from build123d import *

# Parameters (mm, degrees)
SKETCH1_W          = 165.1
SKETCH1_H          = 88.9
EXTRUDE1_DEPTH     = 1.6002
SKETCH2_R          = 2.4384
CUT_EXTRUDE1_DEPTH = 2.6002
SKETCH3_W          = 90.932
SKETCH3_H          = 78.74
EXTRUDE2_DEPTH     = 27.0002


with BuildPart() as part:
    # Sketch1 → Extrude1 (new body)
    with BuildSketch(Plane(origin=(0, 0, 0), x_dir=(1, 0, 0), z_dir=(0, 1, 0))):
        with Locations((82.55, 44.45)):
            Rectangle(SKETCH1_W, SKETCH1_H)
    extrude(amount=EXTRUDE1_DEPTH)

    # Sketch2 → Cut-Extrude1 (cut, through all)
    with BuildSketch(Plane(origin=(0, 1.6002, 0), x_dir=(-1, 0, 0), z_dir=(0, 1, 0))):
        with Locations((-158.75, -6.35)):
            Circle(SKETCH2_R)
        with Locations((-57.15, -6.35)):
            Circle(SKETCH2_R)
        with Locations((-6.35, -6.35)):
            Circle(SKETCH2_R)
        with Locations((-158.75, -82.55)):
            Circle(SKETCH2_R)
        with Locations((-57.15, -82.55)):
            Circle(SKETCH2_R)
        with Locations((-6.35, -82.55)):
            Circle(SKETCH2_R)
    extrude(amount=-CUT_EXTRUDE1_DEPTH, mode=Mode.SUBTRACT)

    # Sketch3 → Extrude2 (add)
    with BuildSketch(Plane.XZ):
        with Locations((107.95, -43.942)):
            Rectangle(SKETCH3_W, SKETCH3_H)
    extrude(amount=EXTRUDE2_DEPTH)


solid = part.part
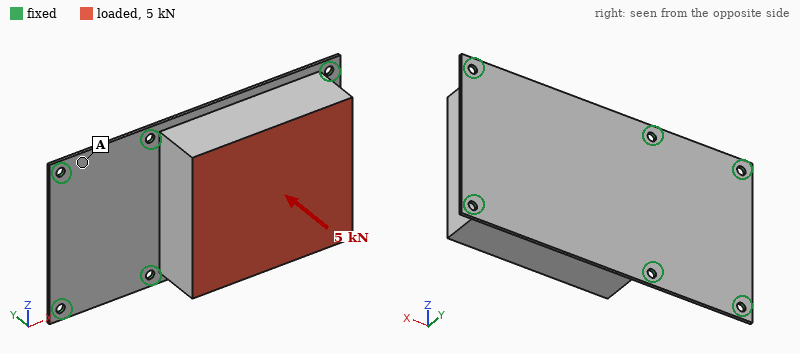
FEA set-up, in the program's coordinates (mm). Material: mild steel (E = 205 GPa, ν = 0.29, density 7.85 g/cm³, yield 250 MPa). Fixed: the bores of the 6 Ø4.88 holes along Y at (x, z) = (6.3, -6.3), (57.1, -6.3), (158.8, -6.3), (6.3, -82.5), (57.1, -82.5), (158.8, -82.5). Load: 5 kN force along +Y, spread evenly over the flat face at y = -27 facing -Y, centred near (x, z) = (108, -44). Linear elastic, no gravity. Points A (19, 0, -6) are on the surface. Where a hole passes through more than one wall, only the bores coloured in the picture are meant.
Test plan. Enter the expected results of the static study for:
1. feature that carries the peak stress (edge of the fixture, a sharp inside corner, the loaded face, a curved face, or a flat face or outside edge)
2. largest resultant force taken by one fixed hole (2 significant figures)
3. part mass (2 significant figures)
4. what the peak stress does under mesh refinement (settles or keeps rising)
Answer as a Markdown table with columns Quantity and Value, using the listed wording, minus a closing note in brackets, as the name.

| Quantity | Value |
|---|---|
| feature that carries the peak stress | edge of the fixture |
| largest resultant force taken by one fixed hole | 1.5 kN |
| part mass | 1.7 kg |
| what the peak stress does under mesh refinement | keeps rising |
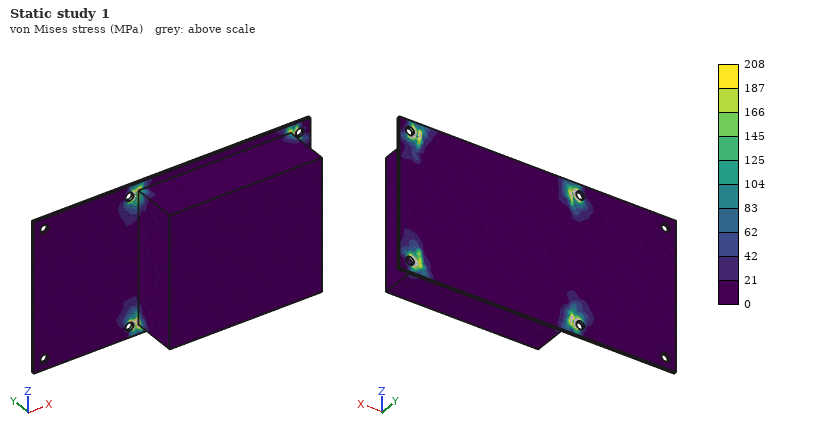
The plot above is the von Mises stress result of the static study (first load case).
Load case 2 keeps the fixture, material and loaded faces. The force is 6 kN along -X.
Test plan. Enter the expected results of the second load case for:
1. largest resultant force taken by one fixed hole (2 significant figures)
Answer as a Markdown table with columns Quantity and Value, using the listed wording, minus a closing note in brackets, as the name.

| Quantity | Value |
|---|---|
| largest resultant force taken by one fixed hole | 1.8 kN |
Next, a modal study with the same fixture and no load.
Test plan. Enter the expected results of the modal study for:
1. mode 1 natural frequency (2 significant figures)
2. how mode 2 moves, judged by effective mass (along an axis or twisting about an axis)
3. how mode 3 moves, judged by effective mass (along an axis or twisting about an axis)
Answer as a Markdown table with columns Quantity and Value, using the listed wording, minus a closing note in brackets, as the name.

| Quantity | Value |
|---|---|
| mode 1 natural frequency | 1600 Hz |
| how mode 2 moves, judged by effective mass | along Y |
| how mode 3 moves, judged by effective mass | along Z |
